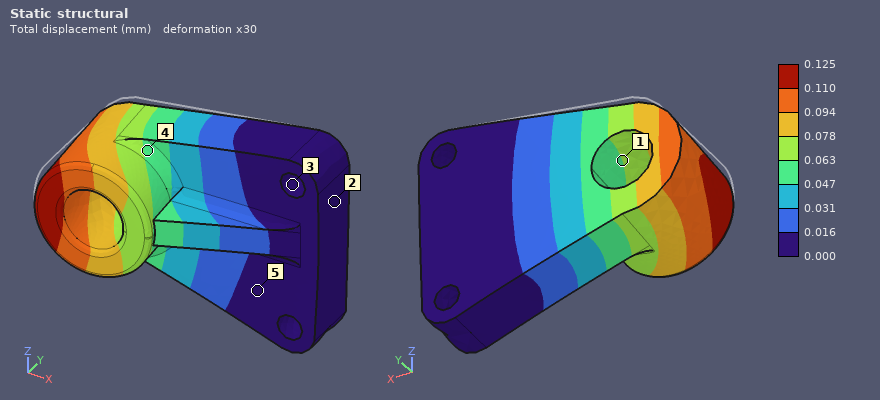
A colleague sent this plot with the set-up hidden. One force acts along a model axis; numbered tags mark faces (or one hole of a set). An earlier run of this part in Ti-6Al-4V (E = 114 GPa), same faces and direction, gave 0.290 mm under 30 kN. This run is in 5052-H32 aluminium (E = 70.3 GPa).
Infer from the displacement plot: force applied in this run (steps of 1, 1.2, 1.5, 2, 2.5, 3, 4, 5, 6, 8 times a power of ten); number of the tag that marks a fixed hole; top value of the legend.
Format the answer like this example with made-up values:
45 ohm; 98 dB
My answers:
8 kN; 3; 0.125 mm
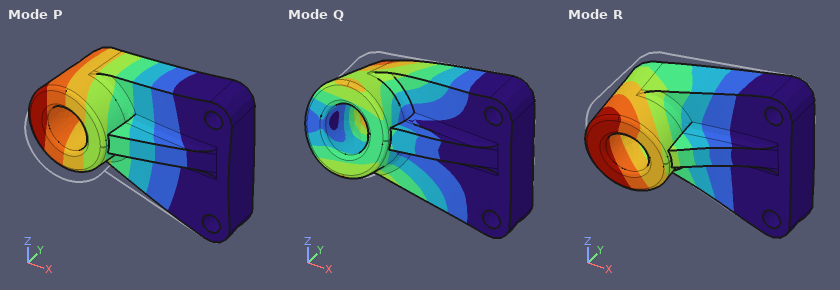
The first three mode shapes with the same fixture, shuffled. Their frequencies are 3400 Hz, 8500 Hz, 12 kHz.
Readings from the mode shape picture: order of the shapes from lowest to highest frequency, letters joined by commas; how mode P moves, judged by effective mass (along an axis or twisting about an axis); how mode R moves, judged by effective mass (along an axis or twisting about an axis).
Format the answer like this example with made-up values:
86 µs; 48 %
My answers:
P, R, Q; along Y; along Z
